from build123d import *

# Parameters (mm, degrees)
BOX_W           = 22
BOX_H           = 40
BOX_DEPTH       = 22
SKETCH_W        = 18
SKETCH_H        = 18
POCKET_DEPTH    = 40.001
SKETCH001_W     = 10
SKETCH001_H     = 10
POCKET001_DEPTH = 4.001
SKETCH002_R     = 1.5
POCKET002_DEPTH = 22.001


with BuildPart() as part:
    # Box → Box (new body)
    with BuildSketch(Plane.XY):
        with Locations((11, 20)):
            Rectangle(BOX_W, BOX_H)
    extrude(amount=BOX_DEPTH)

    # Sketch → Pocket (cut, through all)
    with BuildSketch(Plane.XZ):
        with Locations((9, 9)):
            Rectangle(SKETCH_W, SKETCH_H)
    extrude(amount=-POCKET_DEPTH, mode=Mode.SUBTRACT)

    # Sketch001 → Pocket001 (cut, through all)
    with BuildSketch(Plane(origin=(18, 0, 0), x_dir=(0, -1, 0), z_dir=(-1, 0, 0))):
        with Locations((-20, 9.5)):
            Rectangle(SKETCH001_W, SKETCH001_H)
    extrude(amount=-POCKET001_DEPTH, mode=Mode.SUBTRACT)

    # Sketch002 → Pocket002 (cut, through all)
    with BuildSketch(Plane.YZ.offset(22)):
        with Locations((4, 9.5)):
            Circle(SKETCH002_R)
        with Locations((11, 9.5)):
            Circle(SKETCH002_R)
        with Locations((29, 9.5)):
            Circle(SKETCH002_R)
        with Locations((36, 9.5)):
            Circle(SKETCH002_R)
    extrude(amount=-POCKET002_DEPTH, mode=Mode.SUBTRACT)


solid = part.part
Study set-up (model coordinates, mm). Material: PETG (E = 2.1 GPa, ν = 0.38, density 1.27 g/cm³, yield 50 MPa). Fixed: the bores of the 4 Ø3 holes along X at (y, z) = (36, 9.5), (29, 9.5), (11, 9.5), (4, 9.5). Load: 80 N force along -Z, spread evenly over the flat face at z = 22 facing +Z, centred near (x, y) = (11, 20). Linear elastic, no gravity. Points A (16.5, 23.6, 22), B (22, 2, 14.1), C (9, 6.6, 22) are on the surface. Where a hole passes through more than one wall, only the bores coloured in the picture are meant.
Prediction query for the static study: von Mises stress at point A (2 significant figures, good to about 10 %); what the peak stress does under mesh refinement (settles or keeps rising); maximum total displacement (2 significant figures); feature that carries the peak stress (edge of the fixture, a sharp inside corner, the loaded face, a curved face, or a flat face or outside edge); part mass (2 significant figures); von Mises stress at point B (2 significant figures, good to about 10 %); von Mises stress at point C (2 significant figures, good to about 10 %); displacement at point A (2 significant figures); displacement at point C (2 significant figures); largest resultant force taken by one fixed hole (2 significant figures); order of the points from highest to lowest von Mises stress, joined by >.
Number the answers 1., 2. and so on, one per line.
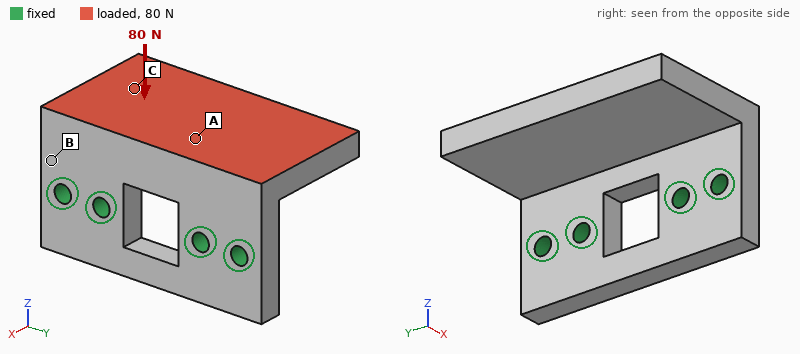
1. 3.5 MPa
2. keeps rising
3. 0.51 mm
4. edge of the fixture
5. 7.5 g
6. 7.7 MPa
7. 1.4 MPa
8. 0.16 mm
9. 0.28 mm
10. 27 N
11. B > A > C
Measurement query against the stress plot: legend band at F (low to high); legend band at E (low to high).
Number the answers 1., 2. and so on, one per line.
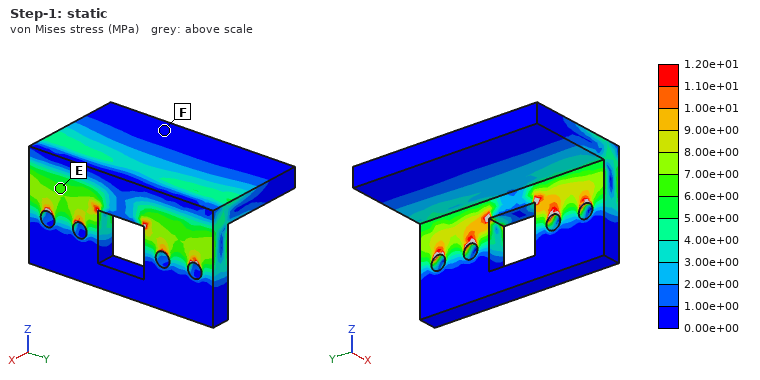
1. 0.00e+00 to 1.00e+00 MPa
2. 6.00e+00 to 7.00e+00 MPa
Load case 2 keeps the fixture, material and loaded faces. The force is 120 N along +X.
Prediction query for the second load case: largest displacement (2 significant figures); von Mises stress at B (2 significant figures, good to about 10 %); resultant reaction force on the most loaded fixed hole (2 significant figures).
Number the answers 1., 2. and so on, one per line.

1. 0.54 mm
2. 11 MPa
3. 31 N
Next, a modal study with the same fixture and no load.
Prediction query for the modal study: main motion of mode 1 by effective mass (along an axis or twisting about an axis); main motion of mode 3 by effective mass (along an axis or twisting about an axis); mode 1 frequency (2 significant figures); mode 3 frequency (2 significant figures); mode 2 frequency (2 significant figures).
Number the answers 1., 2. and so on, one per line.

1. along Z
2. along Y
3. 1100 Hz
4. 3300 Hz
5. 2100 Hz
